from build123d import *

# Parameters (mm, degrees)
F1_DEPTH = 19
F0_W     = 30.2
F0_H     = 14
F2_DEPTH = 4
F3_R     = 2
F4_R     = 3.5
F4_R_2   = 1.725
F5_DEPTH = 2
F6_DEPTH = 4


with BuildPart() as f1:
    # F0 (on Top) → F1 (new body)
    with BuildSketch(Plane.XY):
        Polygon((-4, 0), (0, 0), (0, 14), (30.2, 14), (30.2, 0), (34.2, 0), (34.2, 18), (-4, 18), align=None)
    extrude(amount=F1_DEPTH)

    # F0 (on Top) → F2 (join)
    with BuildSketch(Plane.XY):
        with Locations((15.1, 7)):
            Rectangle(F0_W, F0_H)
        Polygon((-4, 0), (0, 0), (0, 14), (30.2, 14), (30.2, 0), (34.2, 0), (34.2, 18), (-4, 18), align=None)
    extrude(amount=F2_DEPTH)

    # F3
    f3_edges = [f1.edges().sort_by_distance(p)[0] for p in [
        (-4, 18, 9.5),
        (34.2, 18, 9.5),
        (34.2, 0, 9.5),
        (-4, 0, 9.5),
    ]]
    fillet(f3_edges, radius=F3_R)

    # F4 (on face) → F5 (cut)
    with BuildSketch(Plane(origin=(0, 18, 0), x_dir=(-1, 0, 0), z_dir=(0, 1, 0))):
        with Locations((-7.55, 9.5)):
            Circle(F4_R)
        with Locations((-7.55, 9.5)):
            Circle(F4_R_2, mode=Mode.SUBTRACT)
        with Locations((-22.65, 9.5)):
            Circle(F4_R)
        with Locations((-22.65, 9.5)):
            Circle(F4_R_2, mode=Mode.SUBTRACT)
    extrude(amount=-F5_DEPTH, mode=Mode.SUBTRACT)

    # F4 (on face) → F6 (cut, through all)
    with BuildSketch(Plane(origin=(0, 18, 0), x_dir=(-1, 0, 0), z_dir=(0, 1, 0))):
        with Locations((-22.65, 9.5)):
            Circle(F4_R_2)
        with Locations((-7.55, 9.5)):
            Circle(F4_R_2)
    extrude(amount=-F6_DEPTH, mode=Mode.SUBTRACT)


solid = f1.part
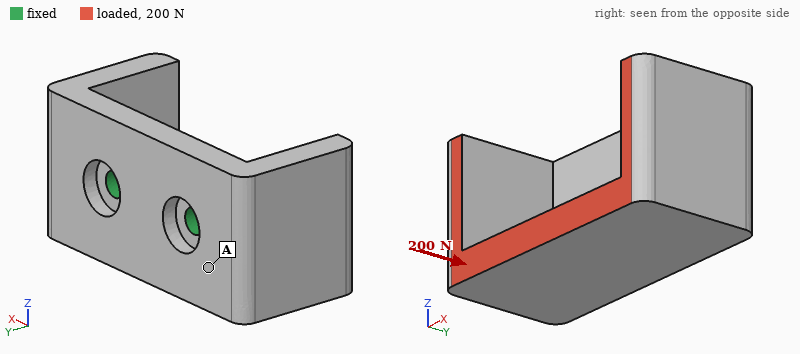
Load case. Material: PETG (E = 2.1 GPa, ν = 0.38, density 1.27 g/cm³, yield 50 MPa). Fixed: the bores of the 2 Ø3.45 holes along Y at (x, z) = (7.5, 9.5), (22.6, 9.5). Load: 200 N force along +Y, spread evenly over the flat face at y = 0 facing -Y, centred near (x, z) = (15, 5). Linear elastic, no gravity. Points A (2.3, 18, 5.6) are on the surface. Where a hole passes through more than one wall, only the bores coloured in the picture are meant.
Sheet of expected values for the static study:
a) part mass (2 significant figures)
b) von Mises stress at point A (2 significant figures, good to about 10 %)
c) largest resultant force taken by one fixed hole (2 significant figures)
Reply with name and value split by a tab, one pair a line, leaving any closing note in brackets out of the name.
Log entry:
part mass	8.2 g
von Mises stress at point A	4.9 MPa
largest resultant force taken by one fixed hole	100 N
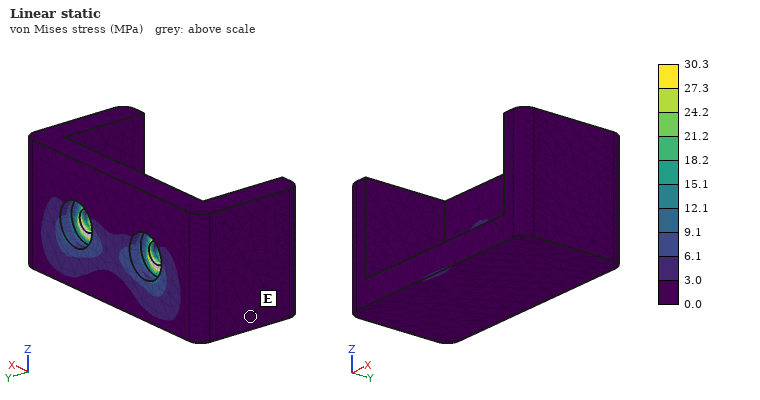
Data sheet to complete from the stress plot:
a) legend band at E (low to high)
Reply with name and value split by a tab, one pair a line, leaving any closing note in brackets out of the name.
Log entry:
legend band at E	0.0 to 3.0 MPa
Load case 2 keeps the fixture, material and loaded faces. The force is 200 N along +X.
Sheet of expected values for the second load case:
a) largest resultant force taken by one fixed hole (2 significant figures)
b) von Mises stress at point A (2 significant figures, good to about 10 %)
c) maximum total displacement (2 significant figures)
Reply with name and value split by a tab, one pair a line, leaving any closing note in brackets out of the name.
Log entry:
largest resultant force taken by one fixed hole	200 N
von Mises stress at point A	5.2 MPa
maximum total displacement	0.52 mm
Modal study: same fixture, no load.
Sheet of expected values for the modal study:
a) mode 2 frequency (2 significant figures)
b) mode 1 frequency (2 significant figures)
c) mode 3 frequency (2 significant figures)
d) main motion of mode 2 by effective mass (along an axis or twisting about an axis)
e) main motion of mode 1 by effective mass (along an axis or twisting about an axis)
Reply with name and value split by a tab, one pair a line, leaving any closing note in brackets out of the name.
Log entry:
mode 2 frequency	1800 Hz
mode 1 frequency	1200 Hz
mode 3 frequency	2600 Hz
main motion of mode 2 by effective mass	along X
main motion of mode 1 by effective mass	along Z
